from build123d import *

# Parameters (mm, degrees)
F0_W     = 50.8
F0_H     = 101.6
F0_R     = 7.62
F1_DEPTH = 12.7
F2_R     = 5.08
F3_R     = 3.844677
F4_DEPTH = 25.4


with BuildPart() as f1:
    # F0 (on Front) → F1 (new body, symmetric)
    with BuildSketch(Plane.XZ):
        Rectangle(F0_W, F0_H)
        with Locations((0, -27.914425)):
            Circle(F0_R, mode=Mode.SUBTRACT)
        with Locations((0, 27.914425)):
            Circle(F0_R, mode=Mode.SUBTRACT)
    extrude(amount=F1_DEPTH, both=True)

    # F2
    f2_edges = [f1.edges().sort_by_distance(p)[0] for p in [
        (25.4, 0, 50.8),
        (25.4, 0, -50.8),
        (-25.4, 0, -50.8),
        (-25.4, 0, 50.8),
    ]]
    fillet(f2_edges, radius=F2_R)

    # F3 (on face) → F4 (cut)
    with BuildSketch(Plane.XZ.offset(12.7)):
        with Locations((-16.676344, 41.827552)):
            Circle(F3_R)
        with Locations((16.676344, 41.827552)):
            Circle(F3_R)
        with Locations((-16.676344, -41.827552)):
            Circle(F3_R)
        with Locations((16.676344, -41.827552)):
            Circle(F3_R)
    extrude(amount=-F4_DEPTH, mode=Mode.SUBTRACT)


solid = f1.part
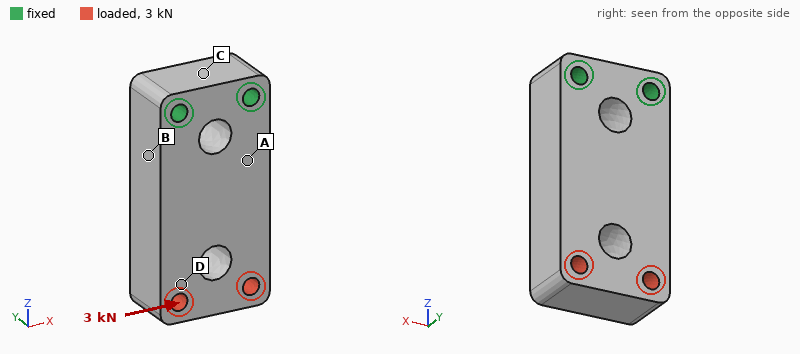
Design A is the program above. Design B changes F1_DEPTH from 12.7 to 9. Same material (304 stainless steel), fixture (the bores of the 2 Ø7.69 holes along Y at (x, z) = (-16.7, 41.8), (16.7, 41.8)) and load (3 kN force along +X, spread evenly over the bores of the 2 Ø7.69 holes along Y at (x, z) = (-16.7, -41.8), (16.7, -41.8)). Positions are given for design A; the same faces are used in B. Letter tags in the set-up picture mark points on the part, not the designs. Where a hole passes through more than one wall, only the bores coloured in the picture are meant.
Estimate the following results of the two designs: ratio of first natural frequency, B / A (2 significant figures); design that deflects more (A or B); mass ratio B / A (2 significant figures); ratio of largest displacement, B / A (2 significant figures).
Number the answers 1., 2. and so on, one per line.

1. 0.73
2. B
3. 0.71
4. 1.4
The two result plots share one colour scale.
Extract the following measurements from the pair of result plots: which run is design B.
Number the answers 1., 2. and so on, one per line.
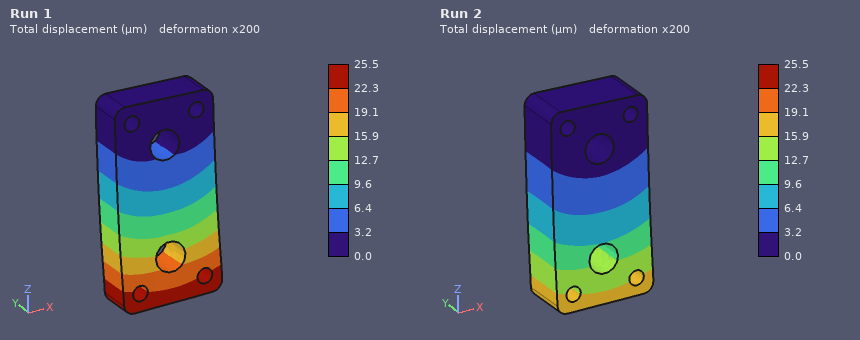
1. Run 1
